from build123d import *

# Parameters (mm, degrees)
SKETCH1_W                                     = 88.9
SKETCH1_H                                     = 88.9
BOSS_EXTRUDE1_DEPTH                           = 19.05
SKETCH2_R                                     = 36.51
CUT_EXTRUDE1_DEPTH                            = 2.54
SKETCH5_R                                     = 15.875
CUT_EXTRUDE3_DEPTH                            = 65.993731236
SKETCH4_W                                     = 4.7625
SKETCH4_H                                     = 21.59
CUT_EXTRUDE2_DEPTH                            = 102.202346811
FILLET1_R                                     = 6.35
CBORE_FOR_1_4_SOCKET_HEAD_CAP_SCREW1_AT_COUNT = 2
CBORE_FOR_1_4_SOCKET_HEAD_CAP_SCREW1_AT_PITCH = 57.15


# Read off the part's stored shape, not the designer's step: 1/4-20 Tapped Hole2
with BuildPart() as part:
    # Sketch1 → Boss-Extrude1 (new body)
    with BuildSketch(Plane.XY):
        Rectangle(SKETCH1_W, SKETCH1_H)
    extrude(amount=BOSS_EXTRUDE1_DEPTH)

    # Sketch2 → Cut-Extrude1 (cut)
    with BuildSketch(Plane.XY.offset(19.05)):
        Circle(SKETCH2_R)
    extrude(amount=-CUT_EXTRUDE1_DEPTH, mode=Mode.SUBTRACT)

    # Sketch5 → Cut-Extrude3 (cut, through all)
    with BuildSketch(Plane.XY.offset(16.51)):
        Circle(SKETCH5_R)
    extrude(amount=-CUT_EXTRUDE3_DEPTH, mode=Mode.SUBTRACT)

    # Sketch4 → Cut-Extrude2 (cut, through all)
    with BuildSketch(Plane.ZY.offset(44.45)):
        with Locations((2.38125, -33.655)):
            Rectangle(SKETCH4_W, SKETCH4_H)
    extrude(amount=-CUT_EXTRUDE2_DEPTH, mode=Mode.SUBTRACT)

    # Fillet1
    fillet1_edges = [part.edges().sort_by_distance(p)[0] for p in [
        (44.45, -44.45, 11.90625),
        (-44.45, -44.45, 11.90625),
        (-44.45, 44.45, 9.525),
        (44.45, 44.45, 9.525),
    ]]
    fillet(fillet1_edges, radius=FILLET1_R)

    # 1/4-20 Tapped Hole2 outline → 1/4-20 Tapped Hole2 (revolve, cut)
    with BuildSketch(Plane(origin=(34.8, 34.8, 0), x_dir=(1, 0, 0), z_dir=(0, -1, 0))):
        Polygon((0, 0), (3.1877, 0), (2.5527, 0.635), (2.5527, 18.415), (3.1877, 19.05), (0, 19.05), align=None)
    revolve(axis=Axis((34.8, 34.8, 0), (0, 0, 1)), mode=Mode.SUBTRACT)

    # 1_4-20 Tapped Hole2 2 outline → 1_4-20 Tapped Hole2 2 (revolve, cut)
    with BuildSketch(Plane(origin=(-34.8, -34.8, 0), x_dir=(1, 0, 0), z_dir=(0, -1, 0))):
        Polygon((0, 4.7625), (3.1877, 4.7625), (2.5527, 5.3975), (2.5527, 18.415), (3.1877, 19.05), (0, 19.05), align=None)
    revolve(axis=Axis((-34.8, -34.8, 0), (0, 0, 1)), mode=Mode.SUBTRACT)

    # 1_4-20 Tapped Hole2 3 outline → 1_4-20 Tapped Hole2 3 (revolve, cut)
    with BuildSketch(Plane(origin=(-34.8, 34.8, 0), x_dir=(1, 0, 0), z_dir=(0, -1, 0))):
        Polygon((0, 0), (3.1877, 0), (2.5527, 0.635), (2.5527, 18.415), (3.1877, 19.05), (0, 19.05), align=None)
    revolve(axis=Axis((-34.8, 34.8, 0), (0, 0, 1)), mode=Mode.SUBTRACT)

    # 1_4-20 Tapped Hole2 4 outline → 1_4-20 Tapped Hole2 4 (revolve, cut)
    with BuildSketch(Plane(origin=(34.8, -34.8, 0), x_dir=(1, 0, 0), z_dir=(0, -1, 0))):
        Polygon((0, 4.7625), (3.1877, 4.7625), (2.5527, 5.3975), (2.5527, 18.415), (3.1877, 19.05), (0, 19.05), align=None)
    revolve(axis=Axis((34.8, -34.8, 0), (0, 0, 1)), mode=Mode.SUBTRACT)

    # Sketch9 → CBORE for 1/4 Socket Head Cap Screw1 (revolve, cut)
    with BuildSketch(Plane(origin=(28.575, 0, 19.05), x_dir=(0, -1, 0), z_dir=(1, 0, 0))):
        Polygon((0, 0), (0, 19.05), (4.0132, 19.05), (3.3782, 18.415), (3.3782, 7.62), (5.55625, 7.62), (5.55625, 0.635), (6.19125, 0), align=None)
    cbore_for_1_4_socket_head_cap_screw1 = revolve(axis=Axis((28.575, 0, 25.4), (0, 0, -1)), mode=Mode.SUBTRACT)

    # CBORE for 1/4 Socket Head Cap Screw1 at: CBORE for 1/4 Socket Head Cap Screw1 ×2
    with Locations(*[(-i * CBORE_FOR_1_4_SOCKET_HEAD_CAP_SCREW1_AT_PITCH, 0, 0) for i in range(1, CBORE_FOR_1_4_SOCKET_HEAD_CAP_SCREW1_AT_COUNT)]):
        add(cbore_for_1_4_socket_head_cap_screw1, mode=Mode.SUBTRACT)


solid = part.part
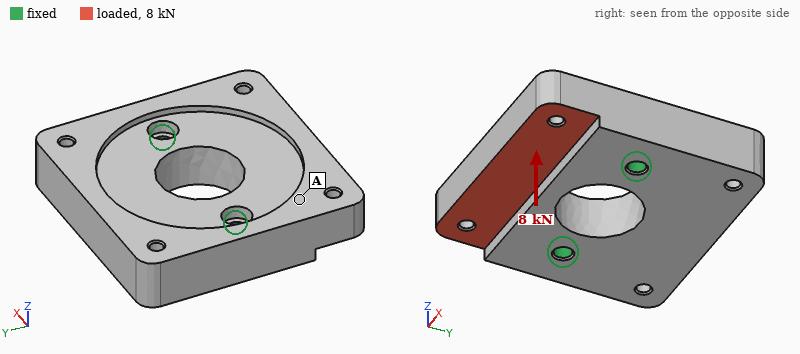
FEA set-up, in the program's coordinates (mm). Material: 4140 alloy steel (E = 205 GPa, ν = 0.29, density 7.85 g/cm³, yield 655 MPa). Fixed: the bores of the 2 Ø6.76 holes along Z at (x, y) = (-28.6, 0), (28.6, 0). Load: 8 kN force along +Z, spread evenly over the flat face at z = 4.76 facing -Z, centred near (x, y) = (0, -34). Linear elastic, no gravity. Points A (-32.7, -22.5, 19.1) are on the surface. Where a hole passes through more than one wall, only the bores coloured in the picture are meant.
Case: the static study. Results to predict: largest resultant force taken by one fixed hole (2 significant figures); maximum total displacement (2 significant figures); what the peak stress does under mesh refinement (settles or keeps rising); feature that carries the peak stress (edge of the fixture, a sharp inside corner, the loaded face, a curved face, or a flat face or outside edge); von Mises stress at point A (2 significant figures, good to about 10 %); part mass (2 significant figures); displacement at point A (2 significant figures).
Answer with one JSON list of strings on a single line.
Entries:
["4.0 kN", "72 µm", "keeps rising", "edge of the fixture", "38 MPa", "890 g", "31 µm"]
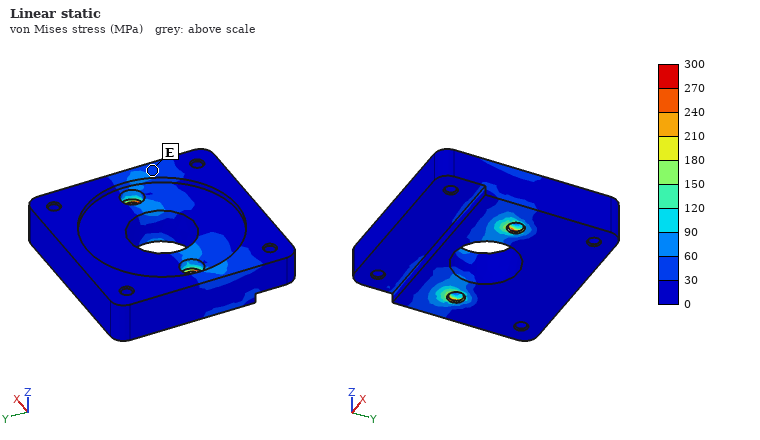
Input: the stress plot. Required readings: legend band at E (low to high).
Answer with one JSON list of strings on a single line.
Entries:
["30 to 60 MPa"]
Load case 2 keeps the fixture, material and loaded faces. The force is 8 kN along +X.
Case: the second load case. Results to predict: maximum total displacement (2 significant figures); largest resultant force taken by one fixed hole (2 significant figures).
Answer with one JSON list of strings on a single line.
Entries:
["12 µm", "5.7 kN"]
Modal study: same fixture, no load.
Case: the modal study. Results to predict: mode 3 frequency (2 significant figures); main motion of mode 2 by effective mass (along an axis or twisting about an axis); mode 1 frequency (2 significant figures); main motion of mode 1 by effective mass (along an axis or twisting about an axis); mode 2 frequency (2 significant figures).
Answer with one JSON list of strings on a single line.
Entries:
["6400 Hz", "along Z", "3200 Hz", "twisting about X", "5400 Hz"]
